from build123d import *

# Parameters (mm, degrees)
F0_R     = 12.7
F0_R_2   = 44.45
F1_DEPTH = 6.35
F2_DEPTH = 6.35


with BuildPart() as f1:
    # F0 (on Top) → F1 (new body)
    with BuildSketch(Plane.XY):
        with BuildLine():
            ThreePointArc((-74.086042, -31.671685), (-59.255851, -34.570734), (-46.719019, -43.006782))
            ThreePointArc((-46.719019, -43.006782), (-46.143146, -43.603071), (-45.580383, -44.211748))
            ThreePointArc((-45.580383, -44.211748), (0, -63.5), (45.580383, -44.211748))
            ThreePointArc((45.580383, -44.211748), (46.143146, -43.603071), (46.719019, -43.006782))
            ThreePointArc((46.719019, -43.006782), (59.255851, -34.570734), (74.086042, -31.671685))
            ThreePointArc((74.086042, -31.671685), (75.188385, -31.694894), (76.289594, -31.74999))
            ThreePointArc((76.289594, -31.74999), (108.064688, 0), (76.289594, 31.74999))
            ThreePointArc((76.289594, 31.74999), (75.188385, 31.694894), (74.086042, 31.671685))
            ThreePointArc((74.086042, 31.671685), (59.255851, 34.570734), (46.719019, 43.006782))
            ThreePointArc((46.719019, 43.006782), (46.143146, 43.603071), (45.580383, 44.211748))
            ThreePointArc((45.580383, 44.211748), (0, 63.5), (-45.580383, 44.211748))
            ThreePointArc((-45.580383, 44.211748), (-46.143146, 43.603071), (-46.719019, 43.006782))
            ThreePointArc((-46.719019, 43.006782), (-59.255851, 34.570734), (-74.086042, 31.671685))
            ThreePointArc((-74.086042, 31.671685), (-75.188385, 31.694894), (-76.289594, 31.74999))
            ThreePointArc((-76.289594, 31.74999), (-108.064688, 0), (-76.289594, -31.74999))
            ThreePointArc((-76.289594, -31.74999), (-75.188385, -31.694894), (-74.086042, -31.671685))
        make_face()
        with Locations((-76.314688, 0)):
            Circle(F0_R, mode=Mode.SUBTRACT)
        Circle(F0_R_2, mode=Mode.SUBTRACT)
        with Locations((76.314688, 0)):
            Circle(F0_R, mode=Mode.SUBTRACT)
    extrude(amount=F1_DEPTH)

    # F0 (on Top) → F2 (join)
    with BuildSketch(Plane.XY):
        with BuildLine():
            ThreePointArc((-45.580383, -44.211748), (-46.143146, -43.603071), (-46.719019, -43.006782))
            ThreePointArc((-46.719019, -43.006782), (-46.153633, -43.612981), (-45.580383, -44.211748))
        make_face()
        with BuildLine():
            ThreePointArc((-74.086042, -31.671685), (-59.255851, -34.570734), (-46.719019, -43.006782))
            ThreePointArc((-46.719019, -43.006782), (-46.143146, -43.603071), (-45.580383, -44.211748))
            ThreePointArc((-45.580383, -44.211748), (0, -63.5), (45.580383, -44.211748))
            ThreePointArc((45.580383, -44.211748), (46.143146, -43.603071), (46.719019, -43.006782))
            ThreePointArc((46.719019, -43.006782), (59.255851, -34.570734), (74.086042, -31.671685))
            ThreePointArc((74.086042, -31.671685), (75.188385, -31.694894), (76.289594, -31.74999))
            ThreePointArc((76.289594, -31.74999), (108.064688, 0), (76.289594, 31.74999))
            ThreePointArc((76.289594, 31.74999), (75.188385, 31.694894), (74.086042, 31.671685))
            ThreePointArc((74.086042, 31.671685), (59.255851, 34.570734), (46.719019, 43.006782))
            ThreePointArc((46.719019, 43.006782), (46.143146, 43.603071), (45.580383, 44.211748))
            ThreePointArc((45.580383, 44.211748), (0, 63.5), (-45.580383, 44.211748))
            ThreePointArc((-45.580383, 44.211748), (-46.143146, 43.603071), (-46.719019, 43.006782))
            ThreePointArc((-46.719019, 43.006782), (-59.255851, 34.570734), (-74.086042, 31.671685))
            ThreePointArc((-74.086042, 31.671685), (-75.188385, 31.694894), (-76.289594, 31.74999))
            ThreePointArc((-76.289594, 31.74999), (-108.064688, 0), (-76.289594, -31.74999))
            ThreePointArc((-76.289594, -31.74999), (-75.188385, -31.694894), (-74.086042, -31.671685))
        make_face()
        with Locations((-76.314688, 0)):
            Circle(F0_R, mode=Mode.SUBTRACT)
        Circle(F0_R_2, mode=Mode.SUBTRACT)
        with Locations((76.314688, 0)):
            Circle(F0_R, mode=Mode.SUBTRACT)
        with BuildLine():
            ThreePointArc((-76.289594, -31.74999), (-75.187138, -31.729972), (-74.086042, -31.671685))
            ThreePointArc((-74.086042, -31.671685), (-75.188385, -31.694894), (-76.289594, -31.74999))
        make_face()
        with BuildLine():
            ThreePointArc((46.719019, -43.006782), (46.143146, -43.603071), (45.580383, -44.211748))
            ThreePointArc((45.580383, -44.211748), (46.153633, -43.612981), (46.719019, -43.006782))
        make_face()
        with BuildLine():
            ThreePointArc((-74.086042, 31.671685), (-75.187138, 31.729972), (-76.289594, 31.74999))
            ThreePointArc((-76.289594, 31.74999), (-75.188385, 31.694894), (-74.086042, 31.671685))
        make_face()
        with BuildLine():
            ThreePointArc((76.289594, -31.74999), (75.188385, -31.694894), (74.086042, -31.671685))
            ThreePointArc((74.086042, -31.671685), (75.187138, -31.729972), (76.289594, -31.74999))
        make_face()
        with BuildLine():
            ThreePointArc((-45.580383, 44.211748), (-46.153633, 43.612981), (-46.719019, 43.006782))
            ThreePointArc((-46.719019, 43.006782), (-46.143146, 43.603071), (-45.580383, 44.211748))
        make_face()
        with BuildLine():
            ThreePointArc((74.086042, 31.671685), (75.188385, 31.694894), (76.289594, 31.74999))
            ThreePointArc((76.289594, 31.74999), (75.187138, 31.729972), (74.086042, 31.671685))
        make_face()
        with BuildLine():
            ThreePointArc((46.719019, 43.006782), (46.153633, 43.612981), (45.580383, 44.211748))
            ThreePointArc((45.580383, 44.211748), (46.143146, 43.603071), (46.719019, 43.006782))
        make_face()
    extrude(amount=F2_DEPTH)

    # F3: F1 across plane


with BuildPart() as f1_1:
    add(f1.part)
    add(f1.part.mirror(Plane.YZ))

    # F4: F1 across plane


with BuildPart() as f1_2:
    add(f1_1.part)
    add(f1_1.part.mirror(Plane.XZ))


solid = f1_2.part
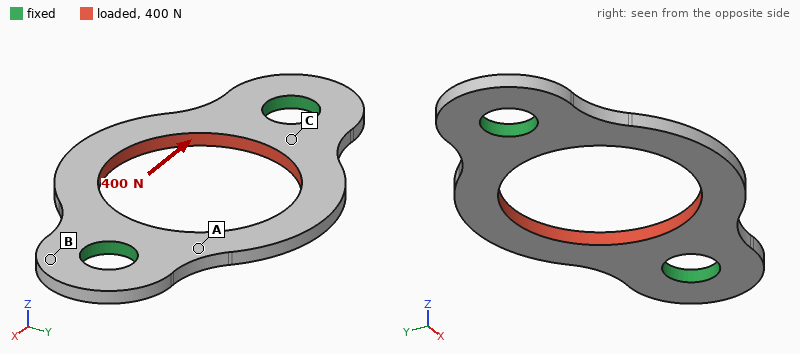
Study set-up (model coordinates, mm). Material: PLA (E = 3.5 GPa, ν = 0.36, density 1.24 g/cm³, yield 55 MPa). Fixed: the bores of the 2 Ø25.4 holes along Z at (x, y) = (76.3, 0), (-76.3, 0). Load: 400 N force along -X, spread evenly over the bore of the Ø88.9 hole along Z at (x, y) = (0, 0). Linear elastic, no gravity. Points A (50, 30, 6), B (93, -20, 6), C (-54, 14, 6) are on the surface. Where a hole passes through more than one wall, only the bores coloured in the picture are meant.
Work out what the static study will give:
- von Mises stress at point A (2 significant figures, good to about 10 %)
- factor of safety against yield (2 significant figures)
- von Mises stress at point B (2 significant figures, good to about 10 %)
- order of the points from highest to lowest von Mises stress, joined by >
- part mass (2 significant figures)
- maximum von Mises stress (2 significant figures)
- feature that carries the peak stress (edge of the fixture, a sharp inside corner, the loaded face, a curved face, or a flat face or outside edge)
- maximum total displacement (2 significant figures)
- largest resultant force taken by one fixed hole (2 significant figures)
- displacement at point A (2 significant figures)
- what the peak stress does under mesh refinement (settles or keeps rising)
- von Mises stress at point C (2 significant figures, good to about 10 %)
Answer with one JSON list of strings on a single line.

["0.70 MPa", "42", "0.25 MPa", "A > C > B", "85 g", "1.3 MPa", "the loaded face", "21 µm", "200 N", "9.1 µm", "settles", "0.49 MPa"]
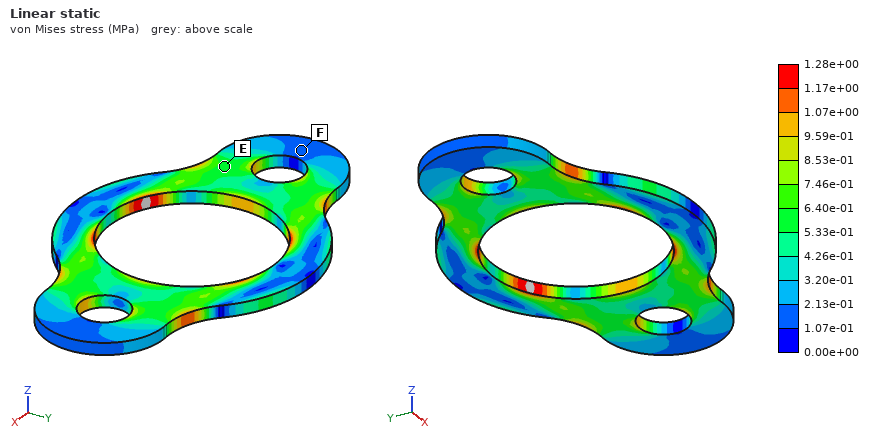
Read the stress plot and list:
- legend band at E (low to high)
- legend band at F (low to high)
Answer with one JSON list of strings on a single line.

["5.33e-01 to 6.40e-01 MPa", "1.07e-01 to 2.13e-01 MPa"]
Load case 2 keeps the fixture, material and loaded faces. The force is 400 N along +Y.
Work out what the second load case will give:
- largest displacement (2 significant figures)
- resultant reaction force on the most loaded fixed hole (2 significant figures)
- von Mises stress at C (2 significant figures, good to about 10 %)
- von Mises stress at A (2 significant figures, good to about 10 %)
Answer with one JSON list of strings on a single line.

["25 µm", "200 N", "0.89 MPa", "0.63 MPa"]
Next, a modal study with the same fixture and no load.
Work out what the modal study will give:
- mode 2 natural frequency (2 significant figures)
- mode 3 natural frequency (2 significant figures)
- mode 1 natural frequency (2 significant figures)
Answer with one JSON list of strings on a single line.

["400 Hz", "1100 Hz", "390 Hz"]
